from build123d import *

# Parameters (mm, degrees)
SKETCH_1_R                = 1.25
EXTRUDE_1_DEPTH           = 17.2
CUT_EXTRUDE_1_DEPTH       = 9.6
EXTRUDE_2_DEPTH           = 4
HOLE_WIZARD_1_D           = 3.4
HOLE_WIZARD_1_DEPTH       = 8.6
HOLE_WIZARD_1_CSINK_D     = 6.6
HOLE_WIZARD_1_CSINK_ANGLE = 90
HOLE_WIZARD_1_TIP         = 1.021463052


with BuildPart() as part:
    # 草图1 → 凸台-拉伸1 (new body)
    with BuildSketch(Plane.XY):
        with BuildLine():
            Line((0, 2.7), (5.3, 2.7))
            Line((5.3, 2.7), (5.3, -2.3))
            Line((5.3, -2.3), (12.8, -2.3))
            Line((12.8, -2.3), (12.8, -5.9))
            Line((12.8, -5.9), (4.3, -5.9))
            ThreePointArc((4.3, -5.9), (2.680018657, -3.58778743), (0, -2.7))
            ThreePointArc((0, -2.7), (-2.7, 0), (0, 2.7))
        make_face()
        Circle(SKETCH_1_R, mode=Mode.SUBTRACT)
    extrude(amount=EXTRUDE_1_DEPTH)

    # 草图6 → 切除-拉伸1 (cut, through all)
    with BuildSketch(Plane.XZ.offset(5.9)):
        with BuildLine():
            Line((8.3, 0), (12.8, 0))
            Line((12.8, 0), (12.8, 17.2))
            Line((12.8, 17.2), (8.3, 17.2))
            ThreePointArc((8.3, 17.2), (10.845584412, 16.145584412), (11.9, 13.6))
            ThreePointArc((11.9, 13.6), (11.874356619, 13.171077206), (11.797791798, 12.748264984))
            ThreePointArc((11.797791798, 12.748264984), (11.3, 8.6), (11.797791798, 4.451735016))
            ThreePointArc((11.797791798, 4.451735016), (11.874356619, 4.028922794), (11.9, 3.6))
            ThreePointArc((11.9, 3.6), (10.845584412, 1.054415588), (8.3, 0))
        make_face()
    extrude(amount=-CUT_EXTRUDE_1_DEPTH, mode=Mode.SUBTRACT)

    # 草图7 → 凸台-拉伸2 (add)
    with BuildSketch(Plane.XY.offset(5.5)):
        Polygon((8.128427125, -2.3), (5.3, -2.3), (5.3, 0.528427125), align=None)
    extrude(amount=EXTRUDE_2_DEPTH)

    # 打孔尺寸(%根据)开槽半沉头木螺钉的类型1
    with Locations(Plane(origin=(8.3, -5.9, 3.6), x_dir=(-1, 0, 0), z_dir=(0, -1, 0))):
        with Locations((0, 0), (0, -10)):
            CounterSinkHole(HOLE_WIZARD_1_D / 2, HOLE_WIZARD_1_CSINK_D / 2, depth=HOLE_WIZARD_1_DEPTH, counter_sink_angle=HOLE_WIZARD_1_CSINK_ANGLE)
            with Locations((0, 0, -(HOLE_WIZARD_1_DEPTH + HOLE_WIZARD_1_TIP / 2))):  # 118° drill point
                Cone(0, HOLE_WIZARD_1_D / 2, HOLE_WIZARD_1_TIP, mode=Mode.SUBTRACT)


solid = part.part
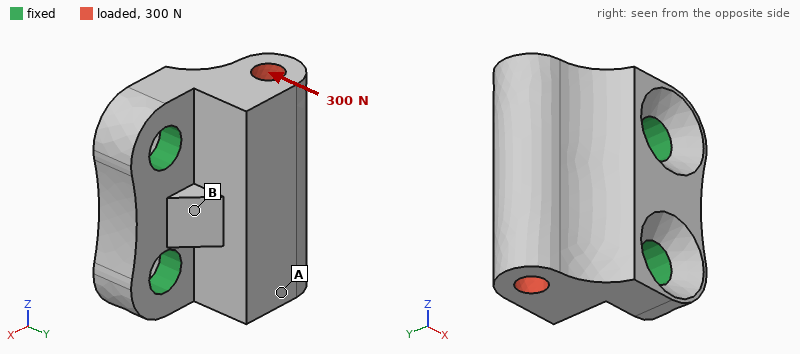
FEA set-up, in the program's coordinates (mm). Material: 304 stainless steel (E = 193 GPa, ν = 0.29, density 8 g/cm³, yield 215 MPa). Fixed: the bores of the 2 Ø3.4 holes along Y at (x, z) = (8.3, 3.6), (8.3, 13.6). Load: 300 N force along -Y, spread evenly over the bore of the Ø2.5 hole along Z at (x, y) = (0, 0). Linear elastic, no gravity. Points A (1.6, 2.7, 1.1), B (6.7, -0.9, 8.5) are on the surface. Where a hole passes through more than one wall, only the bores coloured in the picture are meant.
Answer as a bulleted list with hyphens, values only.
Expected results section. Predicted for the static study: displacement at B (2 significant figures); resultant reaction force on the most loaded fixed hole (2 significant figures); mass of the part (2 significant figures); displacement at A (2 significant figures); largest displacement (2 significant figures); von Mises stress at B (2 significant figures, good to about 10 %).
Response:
- 2.1 µm
- 160 N
- 8.1 g
- 7.7 µm
- 10 µm
- 46 MPa
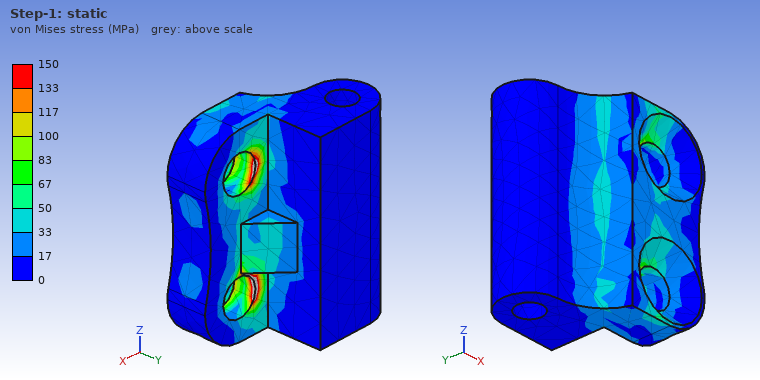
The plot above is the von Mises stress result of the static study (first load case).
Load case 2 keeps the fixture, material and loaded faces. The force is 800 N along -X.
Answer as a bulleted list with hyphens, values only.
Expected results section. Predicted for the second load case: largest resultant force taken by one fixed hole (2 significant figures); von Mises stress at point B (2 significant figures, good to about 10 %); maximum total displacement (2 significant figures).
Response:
- 420 N
- 81 MPa
- 14 µm
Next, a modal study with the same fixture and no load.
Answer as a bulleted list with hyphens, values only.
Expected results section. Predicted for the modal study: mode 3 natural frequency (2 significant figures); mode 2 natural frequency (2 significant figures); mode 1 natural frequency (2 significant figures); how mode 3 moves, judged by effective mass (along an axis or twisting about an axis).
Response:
- 41 kHz
- 34 kHz
- 15 kHz
- along Z
